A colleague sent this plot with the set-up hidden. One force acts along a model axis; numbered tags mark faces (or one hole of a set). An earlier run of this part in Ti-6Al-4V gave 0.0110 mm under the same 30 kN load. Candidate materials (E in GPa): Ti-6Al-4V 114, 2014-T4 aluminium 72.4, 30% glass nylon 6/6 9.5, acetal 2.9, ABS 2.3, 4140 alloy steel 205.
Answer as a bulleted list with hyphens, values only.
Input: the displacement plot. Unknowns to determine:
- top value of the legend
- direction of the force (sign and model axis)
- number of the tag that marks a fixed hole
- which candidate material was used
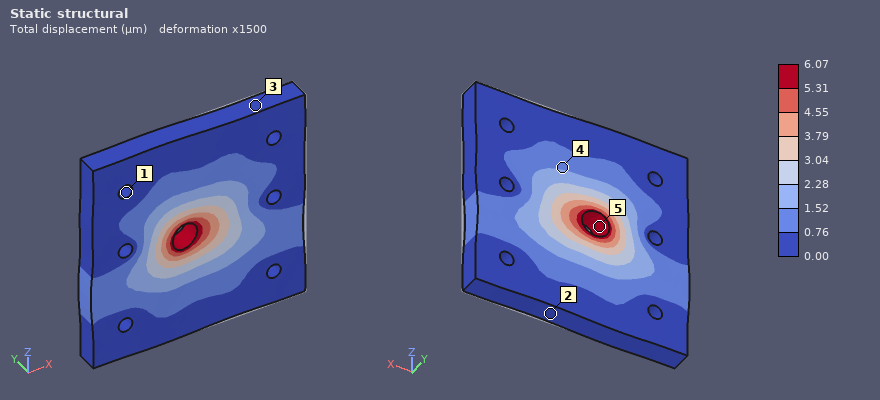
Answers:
- 6.07 µm
- -X
- 1
- 4140 alloy steel
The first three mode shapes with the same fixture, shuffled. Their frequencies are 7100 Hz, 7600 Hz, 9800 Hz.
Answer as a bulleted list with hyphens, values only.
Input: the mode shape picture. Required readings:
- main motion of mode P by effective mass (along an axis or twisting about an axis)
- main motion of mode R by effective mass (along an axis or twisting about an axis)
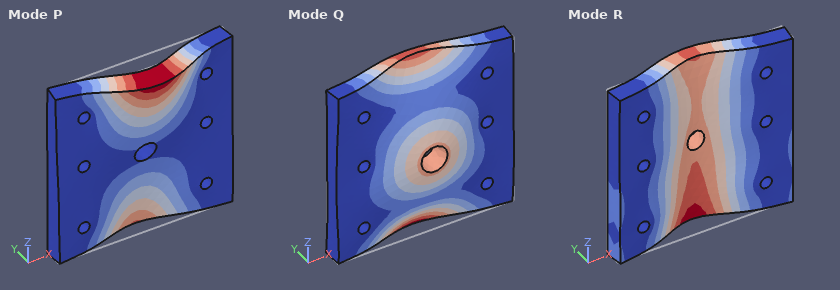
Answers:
- twisting about X
- along Y
